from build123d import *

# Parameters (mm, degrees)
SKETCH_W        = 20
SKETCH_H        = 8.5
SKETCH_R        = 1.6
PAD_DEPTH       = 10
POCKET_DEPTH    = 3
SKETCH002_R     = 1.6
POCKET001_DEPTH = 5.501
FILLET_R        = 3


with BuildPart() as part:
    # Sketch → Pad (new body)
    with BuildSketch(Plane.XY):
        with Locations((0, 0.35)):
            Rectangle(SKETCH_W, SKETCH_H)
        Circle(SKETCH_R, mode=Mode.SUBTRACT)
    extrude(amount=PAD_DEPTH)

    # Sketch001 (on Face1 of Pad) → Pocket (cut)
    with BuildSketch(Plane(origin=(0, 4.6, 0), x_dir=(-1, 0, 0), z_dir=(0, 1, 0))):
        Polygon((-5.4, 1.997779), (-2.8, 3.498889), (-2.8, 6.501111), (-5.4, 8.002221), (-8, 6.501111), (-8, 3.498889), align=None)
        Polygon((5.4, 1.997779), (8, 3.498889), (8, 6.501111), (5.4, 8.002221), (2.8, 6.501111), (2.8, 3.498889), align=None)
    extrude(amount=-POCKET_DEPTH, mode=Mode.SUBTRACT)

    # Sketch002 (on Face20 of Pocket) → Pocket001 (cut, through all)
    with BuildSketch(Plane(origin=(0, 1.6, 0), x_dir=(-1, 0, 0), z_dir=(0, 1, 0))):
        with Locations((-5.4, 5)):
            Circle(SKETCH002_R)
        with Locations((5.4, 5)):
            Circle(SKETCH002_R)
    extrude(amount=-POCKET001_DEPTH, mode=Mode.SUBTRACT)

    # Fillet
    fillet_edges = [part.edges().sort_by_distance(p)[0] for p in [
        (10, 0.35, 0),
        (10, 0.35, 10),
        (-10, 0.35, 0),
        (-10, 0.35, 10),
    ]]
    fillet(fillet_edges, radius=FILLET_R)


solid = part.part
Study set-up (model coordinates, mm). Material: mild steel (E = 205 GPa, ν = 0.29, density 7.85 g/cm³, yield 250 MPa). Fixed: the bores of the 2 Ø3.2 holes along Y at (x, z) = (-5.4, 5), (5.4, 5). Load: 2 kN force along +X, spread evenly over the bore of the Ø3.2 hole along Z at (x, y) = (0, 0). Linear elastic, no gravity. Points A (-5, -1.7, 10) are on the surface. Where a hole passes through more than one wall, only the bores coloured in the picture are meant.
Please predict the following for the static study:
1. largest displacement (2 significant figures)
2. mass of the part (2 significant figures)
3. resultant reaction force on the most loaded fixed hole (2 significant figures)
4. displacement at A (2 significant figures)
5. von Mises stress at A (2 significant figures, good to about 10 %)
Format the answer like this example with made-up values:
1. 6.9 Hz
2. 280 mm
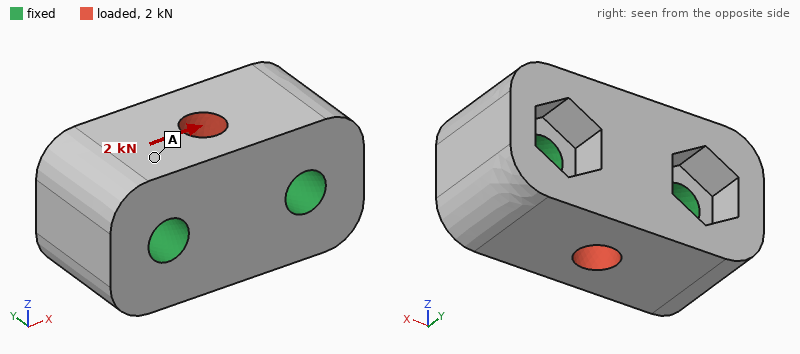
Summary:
1. 0.69 µm
2. 10 g
3. 1.0 kN
4. 0.28 µm
5. 7.9 MPa
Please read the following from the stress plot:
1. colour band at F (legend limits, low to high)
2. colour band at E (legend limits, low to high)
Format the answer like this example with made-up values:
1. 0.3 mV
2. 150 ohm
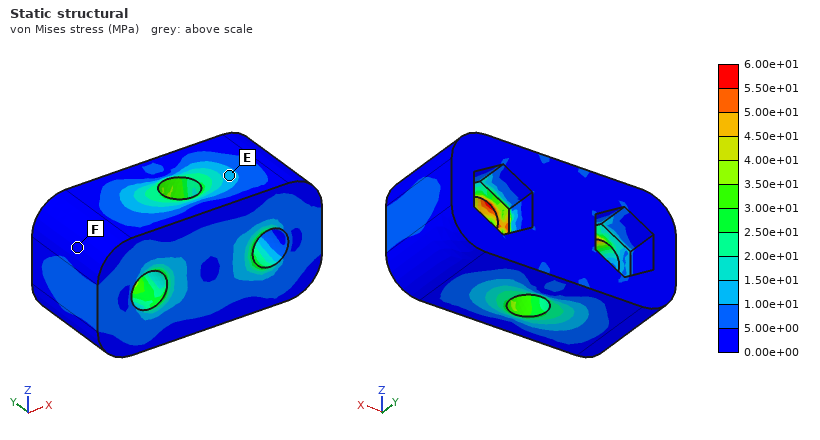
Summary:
1. 0.00e+00 to 5.00e+00 MPa
2. 1.00e+01 to 1.50e+01 MPa
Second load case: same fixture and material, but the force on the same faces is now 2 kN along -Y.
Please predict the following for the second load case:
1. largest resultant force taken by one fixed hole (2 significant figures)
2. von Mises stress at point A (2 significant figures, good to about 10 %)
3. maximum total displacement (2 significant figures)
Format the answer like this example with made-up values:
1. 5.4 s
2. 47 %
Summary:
1. 1.0 kN
2. 11 MPa
3. 1.4 µm
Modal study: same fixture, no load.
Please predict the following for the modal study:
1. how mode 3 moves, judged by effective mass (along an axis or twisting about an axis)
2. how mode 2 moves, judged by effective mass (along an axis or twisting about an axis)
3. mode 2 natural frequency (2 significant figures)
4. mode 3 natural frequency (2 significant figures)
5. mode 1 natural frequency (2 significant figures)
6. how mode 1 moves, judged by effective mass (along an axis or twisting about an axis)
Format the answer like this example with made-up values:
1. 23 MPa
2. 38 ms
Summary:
1. along X
2. twisting about Y
3. 91 kHz
4. 97 kHz
5. 72 kHz
6. along Z
